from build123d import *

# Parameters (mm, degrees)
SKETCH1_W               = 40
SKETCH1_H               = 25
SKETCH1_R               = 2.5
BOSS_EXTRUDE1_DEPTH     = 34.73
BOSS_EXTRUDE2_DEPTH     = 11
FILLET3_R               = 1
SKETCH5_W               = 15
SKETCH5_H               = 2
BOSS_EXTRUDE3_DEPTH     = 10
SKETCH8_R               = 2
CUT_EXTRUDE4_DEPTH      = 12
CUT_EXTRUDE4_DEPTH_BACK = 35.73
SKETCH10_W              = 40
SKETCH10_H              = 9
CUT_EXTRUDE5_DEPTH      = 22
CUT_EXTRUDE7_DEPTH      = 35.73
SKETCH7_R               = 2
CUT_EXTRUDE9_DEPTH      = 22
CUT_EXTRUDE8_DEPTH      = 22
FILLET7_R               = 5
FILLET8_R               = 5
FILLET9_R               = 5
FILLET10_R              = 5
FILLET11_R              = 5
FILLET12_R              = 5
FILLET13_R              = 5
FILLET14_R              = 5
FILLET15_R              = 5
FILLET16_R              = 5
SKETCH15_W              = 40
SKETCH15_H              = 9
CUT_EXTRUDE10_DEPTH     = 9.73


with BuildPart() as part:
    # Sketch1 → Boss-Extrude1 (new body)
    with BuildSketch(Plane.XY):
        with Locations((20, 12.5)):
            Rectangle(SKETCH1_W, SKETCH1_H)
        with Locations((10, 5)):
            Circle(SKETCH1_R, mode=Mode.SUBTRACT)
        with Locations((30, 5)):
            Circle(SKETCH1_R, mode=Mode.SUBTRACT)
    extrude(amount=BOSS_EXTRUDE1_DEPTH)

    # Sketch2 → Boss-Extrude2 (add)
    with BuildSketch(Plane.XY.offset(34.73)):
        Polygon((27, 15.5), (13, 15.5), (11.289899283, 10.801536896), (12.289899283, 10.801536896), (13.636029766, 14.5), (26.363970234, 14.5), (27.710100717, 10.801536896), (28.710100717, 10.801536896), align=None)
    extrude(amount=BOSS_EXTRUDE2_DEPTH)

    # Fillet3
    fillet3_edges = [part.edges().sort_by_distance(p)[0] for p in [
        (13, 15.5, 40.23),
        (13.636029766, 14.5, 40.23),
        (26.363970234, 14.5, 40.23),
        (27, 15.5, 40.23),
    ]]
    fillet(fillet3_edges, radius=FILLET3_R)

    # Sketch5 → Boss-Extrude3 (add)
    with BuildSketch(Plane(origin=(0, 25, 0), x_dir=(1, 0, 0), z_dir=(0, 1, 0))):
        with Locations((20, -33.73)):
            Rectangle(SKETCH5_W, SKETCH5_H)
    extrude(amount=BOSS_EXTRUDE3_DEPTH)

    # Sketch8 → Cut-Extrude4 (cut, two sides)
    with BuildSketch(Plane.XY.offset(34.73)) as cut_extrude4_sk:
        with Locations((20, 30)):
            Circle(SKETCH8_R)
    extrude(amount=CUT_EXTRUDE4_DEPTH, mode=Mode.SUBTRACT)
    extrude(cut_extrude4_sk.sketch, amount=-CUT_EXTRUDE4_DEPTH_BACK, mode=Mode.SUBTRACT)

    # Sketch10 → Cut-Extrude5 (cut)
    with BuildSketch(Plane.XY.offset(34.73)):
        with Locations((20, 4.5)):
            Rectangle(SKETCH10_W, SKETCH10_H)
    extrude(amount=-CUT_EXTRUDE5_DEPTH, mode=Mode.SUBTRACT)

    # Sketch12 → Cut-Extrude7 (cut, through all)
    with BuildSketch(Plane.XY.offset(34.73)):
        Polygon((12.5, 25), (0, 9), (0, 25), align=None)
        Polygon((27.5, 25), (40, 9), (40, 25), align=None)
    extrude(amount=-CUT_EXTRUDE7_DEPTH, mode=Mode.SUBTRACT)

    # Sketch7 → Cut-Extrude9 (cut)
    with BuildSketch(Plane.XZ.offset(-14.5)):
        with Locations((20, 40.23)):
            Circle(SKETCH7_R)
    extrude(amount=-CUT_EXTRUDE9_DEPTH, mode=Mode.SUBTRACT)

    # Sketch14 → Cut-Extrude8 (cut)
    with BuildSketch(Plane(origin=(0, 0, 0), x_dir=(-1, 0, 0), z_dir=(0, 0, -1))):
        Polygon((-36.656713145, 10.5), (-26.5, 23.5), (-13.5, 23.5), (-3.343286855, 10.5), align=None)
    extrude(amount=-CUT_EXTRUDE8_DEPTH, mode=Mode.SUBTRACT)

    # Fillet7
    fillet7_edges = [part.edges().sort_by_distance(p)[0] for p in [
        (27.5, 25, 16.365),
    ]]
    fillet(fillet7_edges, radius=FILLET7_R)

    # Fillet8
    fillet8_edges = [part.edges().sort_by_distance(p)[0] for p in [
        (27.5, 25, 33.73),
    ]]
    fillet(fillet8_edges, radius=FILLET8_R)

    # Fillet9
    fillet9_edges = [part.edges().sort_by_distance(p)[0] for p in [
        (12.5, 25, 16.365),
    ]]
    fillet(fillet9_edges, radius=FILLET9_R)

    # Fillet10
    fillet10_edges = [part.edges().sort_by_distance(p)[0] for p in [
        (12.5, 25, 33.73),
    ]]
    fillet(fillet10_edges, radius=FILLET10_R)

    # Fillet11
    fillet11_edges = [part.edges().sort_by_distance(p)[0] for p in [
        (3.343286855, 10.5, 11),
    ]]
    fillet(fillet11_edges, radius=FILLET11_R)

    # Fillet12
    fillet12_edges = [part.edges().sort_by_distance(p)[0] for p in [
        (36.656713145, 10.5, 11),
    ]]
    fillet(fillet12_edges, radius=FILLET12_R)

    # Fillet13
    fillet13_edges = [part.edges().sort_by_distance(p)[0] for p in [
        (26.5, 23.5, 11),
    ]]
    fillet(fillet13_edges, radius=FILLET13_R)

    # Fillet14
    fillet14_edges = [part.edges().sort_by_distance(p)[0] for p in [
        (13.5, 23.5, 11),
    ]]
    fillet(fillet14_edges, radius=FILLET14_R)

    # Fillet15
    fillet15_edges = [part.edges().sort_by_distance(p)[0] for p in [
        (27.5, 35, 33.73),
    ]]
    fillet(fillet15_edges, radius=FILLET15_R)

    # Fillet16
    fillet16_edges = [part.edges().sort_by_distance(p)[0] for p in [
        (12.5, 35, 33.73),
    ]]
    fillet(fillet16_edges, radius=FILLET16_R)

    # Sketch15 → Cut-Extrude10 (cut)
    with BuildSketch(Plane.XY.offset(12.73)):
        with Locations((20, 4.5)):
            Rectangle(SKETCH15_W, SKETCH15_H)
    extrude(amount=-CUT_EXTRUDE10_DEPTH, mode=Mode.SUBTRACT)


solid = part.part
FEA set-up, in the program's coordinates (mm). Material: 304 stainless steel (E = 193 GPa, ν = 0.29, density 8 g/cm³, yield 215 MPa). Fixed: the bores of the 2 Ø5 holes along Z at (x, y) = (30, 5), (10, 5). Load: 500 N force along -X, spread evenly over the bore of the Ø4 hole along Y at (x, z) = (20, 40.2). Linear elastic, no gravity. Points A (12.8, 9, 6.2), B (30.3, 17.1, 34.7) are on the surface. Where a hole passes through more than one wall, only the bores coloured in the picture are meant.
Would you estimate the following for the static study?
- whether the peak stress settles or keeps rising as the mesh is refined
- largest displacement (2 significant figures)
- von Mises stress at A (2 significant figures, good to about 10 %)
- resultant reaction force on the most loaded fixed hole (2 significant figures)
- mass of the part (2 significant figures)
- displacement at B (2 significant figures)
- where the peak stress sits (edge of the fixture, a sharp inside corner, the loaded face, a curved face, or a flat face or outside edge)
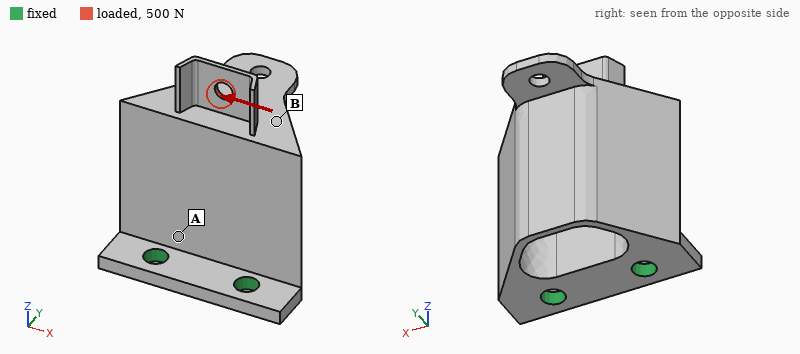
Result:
keeps rising
29 µm
39 MPa
870 N
89 g
15 µm
edge of the fixture
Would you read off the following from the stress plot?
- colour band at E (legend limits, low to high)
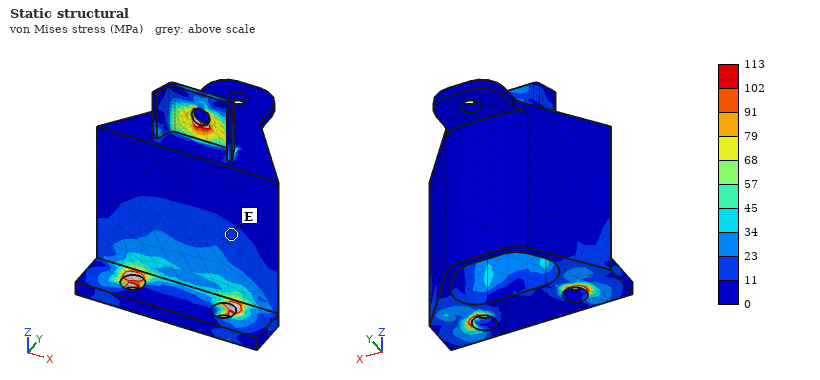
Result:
11 to 23 MPa
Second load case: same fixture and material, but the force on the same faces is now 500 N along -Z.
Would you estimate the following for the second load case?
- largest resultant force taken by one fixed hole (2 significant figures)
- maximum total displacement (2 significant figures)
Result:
250 N
61 µm
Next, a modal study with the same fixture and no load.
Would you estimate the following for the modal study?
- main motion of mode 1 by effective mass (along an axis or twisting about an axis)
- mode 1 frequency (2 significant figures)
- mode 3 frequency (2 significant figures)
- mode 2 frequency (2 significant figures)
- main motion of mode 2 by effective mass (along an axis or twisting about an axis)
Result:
along Y
1100 Hz
7900 Hz
4700 Hz
along X
